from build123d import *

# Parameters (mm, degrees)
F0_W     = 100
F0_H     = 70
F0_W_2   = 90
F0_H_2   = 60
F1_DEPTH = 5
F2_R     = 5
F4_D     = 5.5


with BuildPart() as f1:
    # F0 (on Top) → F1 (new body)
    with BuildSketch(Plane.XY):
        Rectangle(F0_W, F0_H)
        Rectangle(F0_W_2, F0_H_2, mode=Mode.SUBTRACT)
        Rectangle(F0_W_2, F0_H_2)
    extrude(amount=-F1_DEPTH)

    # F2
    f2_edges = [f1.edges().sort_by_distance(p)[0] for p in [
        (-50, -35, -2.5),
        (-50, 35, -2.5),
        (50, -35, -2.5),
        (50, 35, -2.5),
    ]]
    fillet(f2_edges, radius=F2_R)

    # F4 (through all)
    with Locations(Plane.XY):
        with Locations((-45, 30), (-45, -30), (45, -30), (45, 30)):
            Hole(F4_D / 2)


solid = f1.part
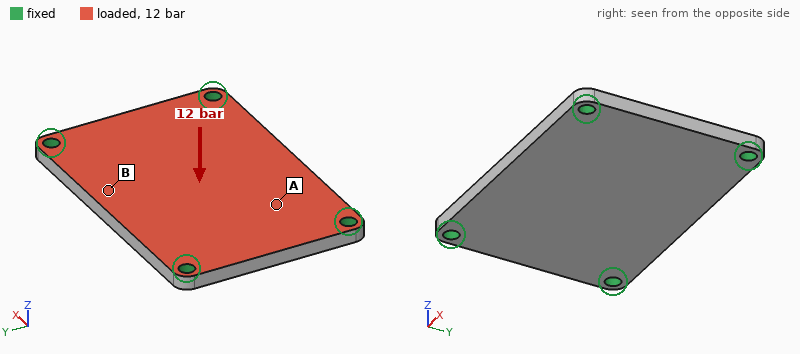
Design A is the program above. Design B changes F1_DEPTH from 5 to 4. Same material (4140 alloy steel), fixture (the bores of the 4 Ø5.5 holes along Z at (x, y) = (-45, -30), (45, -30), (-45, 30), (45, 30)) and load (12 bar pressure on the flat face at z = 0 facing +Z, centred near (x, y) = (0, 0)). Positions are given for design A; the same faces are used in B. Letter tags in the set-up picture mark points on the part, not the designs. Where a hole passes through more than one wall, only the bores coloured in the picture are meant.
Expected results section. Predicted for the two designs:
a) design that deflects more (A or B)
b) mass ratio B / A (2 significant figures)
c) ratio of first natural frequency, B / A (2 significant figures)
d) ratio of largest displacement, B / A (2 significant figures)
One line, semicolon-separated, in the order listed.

B; 0.80; 0.82; 1.9
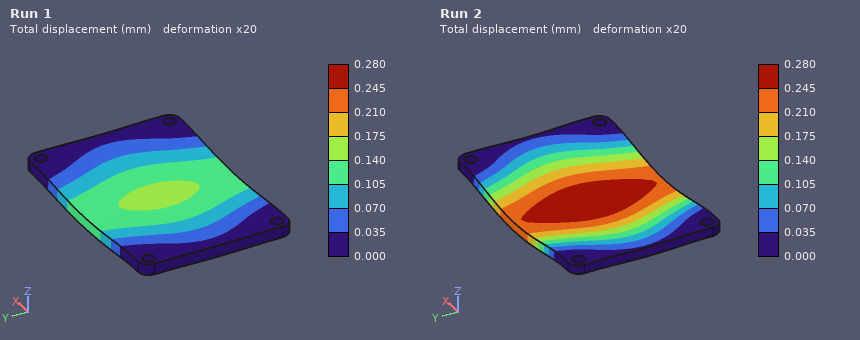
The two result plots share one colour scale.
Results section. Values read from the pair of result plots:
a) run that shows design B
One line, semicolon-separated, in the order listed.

Run 2
